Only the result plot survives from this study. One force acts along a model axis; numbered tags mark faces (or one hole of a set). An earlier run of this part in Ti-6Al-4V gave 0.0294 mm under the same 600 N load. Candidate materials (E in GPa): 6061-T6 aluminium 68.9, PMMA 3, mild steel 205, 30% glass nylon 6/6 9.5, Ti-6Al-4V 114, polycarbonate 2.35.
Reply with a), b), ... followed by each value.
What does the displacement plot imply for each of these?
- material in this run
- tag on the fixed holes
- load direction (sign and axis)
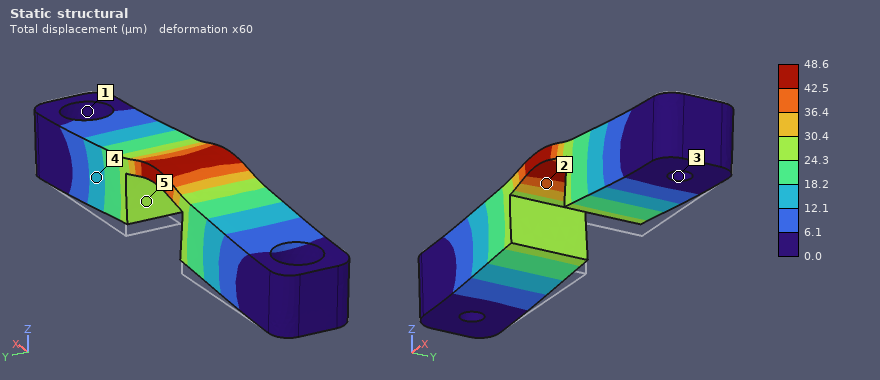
a) 6061-T6 aluminium
b) 3
c) +Z
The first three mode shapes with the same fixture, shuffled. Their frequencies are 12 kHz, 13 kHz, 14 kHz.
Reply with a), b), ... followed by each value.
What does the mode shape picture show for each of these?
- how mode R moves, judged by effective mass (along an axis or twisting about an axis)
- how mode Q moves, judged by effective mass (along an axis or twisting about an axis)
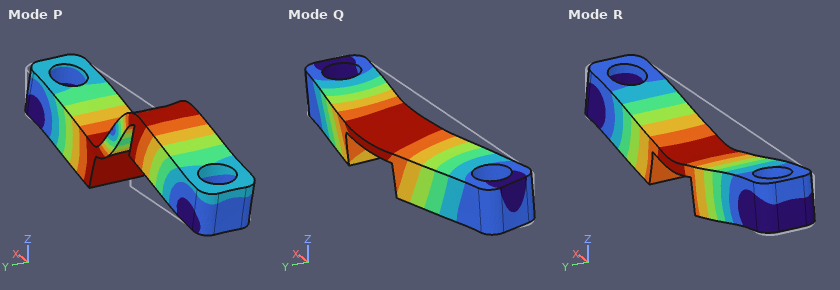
a) along Z
b) along Y
